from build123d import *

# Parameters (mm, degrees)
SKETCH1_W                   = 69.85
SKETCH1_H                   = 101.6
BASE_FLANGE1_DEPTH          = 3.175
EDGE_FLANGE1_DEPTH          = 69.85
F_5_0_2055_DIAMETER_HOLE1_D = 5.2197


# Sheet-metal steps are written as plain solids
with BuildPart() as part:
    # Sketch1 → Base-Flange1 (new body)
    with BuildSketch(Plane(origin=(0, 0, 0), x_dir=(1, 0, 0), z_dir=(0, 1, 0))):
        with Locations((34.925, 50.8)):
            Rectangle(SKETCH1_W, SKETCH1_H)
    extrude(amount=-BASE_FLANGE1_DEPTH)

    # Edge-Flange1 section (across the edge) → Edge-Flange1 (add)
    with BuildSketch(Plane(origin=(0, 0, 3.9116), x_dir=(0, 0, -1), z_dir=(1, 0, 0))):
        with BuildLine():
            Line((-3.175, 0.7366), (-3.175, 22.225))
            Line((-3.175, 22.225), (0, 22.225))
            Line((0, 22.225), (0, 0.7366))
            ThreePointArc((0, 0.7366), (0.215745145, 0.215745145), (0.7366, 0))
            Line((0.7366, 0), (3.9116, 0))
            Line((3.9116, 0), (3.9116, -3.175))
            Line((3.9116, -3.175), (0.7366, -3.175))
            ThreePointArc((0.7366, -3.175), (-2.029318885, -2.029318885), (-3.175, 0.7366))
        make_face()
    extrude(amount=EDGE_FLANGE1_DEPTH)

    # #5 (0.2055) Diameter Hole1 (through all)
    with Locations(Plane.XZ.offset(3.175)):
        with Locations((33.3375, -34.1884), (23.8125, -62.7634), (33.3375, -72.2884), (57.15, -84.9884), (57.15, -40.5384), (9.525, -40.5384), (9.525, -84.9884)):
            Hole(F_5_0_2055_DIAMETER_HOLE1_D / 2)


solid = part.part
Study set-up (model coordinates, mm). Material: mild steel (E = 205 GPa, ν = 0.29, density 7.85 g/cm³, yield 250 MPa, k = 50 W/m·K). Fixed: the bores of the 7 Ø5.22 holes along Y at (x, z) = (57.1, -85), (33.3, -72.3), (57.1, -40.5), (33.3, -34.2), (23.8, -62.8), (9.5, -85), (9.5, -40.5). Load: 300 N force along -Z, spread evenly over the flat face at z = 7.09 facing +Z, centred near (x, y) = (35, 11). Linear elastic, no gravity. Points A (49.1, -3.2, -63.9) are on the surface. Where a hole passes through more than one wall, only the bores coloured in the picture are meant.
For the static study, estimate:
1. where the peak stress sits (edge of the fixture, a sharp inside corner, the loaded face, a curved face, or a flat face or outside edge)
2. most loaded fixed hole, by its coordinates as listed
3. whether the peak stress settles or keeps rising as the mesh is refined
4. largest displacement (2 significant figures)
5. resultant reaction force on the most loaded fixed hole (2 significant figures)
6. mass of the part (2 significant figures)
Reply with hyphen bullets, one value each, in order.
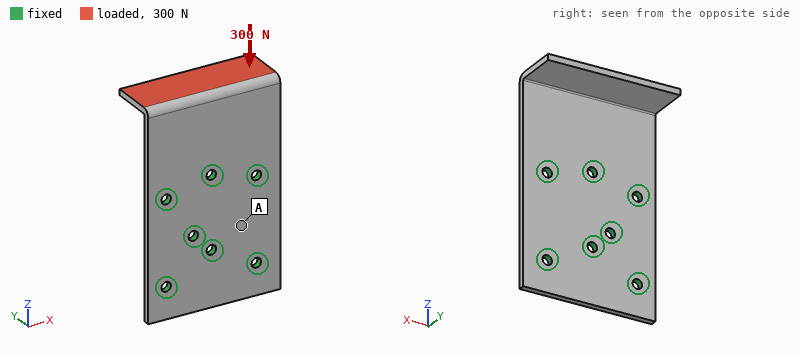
- edge of the fixture
- (33.3, -34.2)
- keeps rising
- 0.14 mm
- 130 N
- 220 g
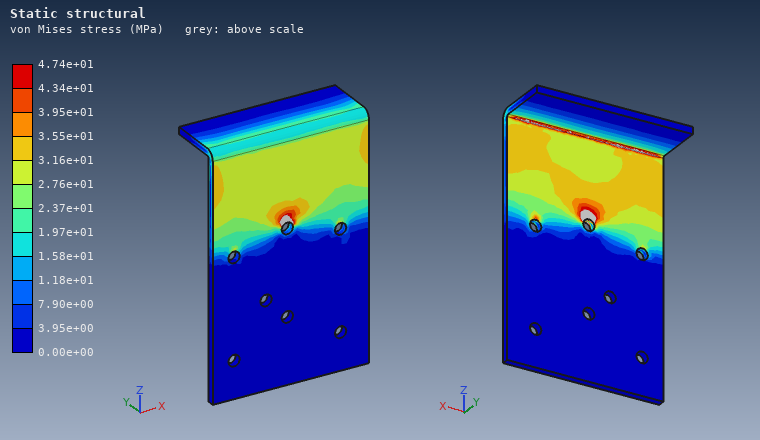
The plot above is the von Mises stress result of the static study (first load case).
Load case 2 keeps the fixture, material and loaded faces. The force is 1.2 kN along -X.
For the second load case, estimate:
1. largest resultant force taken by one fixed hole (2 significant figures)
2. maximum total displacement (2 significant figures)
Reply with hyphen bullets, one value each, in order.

- 960 N
- 0.27 mm
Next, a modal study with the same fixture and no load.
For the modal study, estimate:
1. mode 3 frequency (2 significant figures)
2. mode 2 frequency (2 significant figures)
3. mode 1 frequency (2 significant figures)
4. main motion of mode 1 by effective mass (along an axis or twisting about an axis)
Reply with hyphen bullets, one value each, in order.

- 2900 Hz
- 1400 Hz
- 780 Hz
- along Y
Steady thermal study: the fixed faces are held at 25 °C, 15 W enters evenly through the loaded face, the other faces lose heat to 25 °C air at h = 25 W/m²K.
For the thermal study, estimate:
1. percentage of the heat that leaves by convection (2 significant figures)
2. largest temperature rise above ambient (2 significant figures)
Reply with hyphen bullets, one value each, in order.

- 39 %
- 54 K
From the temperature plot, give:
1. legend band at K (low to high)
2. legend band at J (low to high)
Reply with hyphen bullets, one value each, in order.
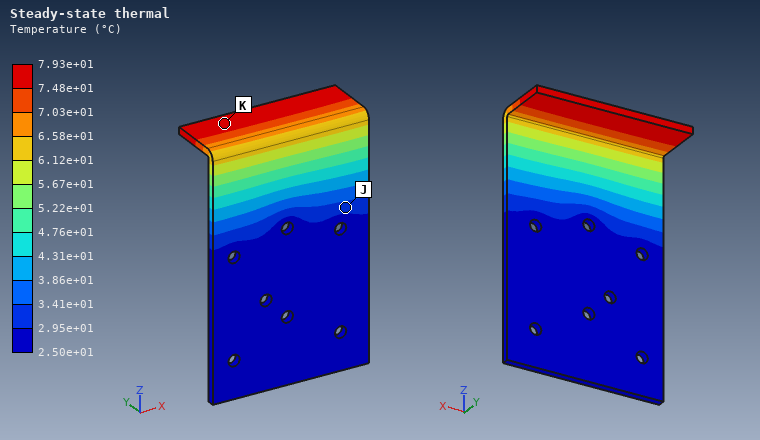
- 7.48e+01 to 7.93e+01 °C
- 2.95e+01 to 3.41e+01 °C
